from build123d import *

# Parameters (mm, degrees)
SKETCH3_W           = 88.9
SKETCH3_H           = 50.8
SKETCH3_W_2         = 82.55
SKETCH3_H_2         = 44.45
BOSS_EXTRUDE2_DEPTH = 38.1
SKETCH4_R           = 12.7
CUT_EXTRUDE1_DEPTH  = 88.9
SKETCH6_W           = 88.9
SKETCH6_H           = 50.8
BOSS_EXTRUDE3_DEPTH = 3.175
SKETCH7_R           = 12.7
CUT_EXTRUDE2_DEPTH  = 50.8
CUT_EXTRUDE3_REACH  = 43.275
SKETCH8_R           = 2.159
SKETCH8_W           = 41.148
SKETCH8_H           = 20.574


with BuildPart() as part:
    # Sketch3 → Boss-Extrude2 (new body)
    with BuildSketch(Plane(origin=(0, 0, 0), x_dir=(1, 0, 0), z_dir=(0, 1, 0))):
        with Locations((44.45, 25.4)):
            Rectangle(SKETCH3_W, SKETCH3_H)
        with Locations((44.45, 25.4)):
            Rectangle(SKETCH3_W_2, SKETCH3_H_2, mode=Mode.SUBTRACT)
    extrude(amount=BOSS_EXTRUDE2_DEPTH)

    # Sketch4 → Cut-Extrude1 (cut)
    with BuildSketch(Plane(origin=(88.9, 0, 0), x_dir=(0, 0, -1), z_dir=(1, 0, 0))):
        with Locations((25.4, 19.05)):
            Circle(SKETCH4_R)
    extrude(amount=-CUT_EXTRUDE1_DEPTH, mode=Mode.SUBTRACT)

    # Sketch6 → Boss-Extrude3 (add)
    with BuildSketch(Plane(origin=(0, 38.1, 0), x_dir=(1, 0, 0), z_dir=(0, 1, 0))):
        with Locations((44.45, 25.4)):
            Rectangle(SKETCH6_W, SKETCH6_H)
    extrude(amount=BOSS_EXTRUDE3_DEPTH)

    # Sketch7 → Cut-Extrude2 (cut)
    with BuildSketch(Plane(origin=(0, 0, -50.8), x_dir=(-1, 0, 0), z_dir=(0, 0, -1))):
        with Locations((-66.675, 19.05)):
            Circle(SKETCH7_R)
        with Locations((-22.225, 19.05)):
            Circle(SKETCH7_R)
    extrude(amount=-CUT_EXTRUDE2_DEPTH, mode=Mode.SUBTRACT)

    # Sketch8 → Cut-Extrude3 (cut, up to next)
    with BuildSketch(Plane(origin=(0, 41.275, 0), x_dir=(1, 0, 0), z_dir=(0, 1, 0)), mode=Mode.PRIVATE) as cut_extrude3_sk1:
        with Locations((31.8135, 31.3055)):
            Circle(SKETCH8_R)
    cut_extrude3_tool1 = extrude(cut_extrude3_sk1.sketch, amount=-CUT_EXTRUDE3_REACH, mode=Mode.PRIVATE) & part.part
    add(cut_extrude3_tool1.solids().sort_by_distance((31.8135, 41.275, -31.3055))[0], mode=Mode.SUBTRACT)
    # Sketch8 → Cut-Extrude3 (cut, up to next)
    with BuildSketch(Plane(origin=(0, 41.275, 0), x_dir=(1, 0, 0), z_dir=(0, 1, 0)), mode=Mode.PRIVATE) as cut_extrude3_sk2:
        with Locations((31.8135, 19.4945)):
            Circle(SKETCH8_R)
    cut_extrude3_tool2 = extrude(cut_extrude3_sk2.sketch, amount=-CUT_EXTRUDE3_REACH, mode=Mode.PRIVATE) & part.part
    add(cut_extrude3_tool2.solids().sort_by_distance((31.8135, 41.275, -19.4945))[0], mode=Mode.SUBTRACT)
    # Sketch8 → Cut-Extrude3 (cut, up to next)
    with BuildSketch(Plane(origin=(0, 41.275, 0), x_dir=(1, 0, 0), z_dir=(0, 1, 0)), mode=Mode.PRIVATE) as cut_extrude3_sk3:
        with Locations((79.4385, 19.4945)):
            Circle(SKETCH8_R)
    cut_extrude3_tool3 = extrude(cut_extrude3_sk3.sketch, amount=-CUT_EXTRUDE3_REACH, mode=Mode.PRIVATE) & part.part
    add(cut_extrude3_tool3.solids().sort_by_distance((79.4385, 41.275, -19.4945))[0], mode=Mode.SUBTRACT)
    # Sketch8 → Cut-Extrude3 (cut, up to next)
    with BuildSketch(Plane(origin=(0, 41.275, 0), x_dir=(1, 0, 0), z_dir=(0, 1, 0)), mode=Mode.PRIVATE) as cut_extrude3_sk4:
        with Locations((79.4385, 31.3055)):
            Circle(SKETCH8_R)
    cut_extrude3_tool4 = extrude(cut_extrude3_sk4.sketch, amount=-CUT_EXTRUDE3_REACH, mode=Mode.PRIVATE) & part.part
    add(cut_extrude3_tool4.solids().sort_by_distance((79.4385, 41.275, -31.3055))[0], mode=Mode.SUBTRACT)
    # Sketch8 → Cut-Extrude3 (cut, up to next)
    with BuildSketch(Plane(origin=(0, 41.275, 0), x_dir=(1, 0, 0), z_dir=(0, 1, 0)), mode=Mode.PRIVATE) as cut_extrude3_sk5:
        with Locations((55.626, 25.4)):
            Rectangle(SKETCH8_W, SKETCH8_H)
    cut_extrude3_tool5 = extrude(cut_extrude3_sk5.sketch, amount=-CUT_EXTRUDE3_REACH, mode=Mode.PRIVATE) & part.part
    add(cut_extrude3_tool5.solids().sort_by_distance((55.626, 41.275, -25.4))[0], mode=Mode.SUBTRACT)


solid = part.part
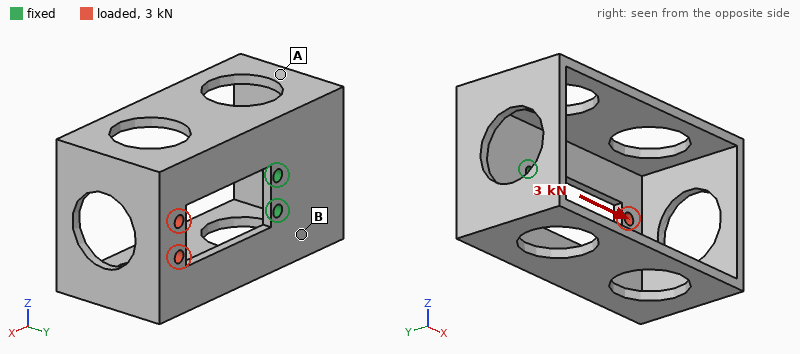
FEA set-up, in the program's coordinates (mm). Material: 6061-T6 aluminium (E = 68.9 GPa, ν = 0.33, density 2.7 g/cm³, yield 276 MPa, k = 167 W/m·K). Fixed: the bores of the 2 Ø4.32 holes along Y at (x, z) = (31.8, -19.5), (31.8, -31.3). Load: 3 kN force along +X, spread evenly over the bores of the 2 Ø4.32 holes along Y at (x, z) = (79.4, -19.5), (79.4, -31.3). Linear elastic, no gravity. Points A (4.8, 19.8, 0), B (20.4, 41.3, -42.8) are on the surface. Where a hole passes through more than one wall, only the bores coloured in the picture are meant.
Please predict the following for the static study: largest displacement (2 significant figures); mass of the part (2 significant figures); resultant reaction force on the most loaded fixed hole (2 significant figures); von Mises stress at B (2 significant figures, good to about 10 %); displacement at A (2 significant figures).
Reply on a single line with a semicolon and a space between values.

73 µm; 92 g; 1.7 kN; 22 MPa; 17 µm
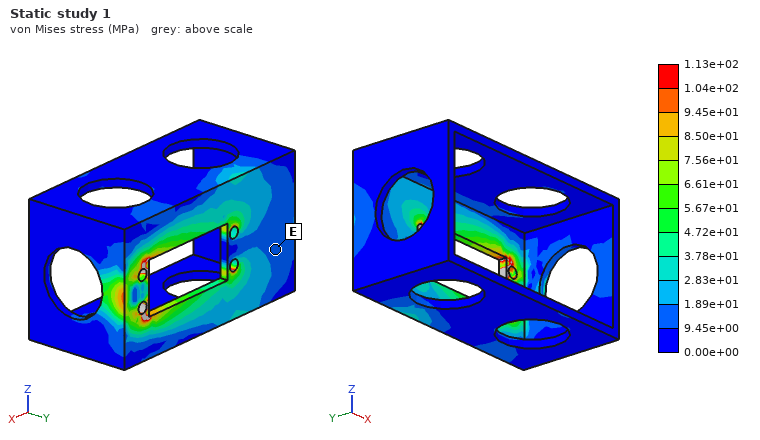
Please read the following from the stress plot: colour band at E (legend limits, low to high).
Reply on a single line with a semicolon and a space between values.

9.45e+00 to 1.89e+01 MPa
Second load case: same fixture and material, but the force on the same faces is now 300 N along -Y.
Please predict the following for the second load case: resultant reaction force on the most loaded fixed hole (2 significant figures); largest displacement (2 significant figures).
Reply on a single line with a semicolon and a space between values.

200 N; 1.1 mm
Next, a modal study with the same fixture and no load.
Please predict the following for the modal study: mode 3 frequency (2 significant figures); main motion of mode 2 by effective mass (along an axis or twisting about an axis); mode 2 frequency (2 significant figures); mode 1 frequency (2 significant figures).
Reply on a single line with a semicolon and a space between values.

1300 Hz; along Z; 820 Hz; 420 Hz
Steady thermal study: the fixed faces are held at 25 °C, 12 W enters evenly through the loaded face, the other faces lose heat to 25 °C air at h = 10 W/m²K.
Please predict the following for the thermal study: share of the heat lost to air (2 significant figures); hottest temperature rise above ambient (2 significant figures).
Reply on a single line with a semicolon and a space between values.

23 %; 31 K
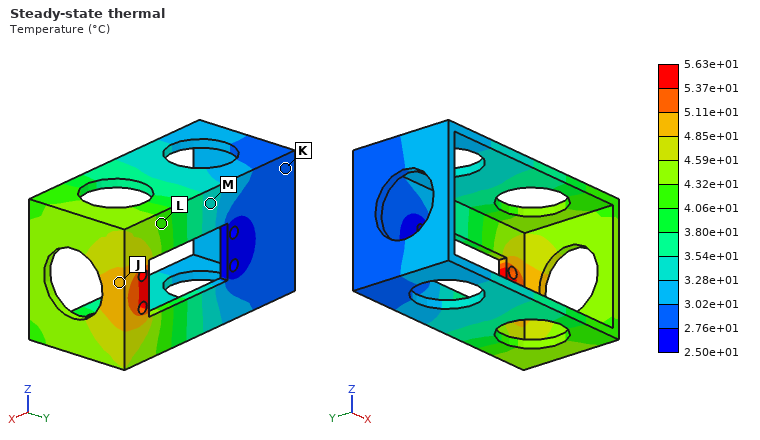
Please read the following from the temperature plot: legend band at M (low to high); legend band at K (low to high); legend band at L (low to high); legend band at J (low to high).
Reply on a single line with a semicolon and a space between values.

3.28e+01 to 3.54e+01 °C; 2.76e+01 to 3.02e+01 °C; 4.06e+01 to 4.32e+01 °C; 4.85e+01 to 5.11e+01 °C
